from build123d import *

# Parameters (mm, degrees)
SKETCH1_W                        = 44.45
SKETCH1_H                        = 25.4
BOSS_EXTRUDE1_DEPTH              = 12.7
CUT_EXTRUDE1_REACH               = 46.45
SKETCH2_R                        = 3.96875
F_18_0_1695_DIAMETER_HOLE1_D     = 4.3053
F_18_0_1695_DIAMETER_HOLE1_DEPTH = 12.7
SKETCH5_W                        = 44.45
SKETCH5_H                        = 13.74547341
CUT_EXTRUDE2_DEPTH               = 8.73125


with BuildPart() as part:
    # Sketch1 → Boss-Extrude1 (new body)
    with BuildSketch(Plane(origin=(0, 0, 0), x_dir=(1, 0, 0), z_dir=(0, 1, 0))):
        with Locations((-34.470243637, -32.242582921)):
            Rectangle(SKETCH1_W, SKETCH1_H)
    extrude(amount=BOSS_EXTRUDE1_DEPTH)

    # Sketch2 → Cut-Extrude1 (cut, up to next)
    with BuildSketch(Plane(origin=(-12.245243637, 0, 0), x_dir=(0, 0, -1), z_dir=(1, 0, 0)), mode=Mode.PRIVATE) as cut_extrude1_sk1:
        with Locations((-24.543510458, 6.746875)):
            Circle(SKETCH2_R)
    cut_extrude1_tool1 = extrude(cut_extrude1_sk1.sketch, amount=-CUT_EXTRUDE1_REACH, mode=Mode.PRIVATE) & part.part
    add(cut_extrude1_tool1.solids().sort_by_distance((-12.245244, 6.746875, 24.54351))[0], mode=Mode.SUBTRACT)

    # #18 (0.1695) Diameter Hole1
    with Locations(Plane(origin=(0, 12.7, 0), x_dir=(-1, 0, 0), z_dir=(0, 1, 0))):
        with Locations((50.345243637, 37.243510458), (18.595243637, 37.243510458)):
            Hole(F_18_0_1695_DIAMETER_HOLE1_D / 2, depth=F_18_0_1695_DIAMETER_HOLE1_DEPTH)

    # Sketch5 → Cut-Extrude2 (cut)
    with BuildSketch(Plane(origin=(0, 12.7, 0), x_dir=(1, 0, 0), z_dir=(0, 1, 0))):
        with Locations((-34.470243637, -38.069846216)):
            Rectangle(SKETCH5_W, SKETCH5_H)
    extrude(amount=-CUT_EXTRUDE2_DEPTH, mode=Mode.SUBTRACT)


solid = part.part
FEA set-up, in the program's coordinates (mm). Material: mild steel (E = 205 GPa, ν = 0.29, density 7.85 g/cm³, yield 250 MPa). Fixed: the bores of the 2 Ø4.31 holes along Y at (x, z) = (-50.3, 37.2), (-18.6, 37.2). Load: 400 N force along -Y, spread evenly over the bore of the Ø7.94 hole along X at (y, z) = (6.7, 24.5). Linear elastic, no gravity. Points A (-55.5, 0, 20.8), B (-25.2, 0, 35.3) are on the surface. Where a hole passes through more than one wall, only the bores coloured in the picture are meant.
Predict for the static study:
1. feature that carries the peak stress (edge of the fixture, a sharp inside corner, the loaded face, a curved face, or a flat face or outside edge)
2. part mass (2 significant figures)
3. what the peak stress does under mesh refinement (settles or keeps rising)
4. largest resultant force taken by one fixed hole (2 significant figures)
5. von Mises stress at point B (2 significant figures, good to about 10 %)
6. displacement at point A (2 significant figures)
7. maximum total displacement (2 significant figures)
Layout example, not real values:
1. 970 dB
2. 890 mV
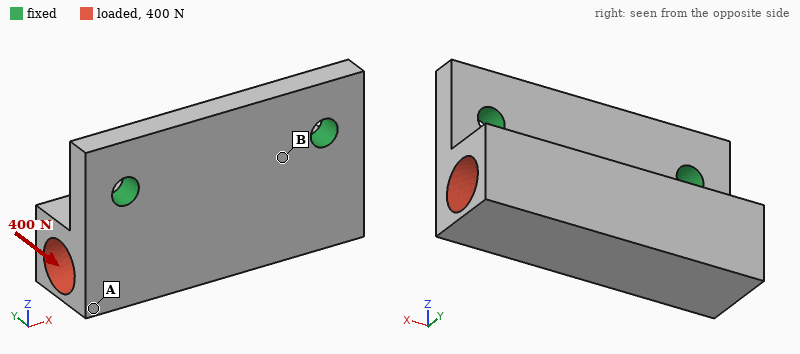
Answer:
1. edge of the fixture
2. 53 g
3. keeps rising
4. 200 N
5. 19 MPa
6. 9.3 µm
7. 13 µm
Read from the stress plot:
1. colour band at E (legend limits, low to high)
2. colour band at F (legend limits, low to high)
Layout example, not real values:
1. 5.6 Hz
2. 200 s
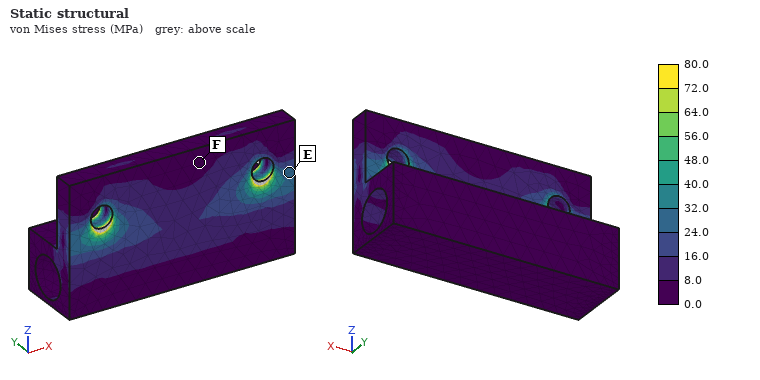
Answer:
1. 24.0 to 32.0 MPa
2. 0.0 to 8.0 MPa
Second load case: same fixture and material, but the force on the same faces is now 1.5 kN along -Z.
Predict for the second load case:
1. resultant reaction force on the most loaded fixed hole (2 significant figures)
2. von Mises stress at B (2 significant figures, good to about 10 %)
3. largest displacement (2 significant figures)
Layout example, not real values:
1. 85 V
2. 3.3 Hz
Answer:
1. 760 N
2. 32 MPa
3. 26 µm
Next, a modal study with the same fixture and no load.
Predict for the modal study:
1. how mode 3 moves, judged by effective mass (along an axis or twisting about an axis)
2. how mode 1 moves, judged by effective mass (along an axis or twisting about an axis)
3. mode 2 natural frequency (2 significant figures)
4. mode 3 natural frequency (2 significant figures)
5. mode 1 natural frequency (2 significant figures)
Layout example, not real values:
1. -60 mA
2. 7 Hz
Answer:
1. along Y
2. along Y
3. 15 kHz
4. 20 kHz
5. 5700 Hz
